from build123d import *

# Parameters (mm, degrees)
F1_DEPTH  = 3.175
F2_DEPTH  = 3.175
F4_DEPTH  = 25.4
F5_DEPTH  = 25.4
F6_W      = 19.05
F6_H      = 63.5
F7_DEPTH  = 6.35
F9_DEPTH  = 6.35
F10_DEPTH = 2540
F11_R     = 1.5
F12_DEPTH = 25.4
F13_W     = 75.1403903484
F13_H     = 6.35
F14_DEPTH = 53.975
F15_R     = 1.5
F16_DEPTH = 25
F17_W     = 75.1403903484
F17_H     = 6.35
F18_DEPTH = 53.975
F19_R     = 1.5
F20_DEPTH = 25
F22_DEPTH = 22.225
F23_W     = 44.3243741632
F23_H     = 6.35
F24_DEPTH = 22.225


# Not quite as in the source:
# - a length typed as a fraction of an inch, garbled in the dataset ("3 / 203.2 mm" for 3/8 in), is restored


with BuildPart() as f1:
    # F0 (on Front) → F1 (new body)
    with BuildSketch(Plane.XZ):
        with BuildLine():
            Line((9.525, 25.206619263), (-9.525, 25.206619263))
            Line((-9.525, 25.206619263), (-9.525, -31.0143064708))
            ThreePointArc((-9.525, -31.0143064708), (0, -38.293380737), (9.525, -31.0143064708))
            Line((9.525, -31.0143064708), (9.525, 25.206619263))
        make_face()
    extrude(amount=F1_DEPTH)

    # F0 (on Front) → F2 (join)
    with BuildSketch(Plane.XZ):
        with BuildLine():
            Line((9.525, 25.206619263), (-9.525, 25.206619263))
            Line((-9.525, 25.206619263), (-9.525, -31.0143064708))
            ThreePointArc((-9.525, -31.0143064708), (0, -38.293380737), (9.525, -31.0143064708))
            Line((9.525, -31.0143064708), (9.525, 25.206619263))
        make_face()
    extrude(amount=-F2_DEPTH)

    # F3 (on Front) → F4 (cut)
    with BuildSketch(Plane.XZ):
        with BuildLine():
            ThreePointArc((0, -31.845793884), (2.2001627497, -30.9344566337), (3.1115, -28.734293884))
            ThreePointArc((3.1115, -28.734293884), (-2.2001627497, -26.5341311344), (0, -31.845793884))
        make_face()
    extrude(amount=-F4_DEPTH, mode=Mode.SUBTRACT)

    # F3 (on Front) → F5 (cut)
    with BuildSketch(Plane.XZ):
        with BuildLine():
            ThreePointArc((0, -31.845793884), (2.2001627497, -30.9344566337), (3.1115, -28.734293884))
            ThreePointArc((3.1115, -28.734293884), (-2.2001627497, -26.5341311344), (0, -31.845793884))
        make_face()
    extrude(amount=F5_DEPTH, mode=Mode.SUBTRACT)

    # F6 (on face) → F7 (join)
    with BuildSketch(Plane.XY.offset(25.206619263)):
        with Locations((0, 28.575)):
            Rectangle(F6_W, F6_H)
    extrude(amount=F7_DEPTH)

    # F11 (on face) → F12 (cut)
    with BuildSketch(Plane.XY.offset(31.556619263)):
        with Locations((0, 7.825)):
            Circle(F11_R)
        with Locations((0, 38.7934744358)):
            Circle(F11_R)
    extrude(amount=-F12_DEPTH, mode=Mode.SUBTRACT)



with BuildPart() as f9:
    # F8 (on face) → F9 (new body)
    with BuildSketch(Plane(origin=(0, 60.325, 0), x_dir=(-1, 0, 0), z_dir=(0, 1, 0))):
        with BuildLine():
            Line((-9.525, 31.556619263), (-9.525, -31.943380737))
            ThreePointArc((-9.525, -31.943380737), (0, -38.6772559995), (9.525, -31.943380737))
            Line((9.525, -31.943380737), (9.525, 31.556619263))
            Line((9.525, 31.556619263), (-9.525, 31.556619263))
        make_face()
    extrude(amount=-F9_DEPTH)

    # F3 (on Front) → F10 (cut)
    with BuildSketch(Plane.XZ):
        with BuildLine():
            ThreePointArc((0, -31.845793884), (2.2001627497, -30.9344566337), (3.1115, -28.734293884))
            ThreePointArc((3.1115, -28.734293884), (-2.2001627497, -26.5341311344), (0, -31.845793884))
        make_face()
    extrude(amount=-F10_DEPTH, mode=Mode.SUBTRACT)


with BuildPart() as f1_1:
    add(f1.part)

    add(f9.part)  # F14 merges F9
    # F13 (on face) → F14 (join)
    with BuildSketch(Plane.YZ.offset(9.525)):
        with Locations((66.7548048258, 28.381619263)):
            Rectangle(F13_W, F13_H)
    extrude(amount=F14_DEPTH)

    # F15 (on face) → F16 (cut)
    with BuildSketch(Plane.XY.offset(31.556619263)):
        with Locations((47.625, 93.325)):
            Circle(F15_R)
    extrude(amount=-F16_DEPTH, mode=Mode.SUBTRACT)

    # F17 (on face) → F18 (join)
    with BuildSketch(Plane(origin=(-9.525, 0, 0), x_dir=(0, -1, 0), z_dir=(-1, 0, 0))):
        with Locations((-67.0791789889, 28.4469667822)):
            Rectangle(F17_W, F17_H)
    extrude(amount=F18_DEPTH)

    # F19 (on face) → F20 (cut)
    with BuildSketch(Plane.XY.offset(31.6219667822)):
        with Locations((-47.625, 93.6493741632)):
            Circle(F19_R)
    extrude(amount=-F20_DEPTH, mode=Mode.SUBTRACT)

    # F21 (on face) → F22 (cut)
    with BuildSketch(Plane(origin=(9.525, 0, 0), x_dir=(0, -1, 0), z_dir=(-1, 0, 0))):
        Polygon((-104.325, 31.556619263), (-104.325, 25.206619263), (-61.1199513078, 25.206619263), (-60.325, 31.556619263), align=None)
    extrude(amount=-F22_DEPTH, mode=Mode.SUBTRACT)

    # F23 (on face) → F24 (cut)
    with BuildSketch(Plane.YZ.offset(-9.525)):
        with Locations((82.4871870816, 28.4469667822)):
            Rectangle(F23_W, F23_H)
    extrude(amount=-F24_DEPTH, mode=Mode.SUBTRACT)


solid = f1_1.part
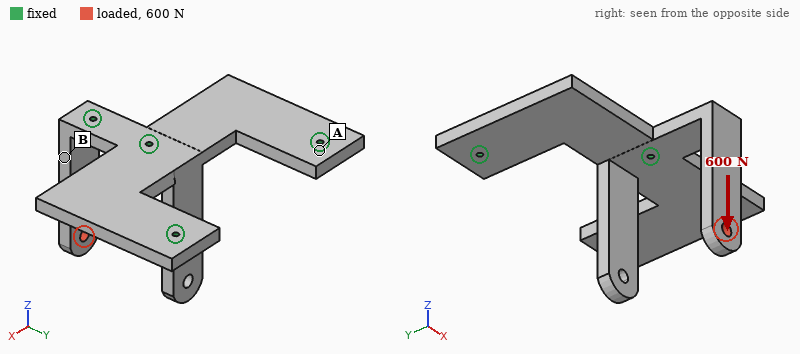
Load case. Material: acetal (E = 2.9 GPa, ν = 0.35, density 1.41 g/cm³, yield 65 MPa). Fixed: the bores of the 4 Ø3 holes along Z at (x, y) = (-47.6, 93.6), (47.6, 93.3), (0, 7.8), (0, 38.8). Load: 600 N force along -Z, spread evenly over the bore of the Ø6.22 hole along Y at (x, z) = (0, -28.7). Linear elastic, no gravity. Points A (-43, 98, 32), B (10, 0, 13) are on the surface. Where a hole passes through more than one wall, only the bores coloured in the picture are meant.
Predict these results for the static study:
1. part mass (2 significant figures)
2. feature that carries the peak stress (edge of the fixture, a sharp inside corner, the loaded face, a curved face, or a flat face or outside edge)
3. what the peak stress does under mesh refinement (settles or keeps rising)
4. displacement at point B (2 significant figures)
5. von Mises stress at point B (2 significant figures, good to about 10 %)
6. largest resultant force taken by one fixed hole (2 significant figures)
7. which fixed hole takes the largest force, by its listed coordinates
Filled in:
86 g
edge of the fixture
keeps rising
0.38 mm
4.8 MPa
650 N
(0, 7.8)
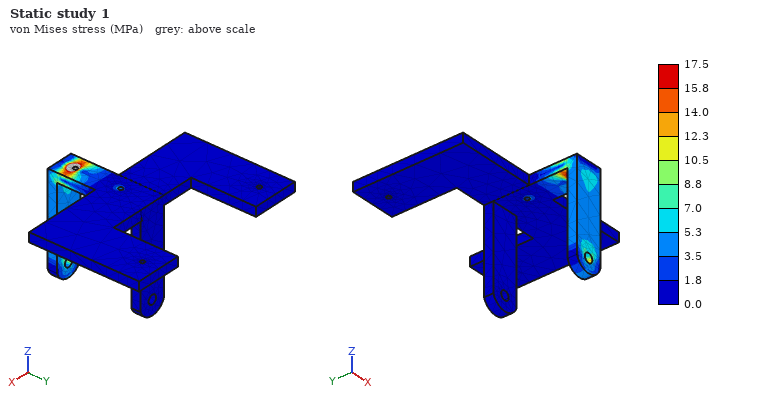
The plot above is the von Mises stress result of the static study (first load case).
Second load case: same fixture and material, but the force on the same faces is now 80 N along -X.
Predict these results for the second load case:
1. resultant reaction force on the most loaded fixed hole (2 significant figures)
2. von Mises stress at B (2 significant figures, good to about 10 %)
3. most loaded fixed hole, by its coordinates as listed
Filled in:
98 N
8.7 MPa
(0, 7.8)
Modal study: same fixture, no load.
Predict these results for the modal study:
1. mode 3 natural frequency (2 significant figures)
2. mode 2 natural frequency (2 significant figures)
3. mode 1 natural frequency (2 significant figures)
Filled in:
500 Hz
300 Hz
300 Hz
